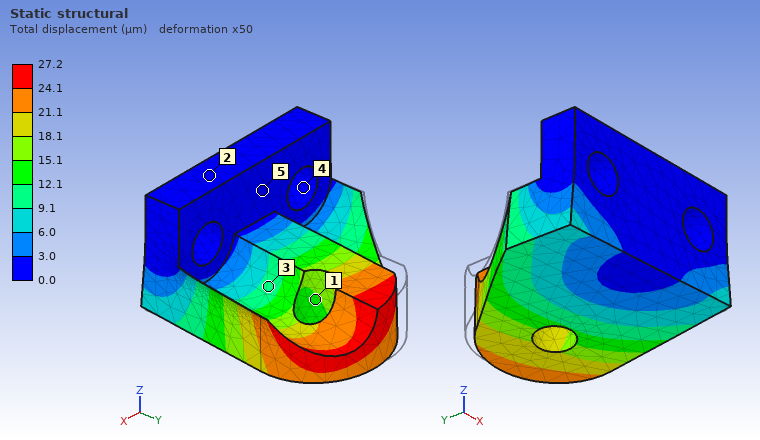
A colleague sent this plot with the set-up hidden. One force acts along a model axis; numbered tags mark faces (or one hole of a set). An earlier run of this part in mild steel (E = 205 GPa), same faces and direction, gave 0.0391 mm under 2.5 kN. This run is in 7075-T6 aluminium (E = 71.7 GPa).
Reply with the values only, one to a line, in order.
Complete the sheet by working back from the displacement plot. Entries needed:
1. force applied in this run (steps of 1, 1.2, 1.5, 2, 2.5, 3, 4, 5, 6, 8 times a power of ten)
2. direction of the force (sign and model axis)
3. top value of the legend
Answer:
600 N
+X
27.2 µm
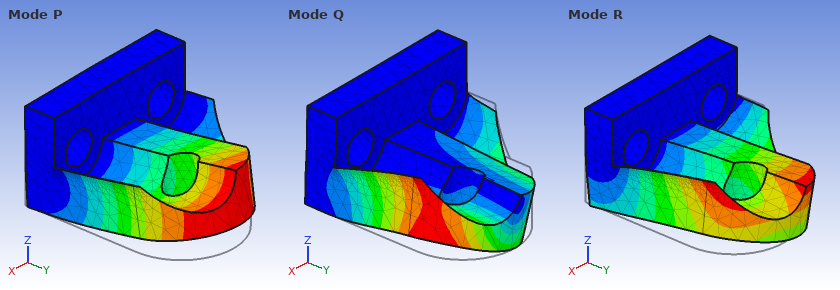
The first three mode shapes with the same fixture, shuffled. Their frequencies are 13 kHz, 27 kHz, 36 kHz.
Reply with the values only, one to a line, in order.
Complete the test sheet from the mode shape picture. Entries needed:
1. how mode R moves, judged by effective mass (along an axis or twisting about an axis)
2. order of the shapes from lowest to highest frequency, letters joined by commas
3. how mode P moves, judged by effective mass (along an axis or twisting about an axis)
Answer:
along X
P, R, Q
along Z
